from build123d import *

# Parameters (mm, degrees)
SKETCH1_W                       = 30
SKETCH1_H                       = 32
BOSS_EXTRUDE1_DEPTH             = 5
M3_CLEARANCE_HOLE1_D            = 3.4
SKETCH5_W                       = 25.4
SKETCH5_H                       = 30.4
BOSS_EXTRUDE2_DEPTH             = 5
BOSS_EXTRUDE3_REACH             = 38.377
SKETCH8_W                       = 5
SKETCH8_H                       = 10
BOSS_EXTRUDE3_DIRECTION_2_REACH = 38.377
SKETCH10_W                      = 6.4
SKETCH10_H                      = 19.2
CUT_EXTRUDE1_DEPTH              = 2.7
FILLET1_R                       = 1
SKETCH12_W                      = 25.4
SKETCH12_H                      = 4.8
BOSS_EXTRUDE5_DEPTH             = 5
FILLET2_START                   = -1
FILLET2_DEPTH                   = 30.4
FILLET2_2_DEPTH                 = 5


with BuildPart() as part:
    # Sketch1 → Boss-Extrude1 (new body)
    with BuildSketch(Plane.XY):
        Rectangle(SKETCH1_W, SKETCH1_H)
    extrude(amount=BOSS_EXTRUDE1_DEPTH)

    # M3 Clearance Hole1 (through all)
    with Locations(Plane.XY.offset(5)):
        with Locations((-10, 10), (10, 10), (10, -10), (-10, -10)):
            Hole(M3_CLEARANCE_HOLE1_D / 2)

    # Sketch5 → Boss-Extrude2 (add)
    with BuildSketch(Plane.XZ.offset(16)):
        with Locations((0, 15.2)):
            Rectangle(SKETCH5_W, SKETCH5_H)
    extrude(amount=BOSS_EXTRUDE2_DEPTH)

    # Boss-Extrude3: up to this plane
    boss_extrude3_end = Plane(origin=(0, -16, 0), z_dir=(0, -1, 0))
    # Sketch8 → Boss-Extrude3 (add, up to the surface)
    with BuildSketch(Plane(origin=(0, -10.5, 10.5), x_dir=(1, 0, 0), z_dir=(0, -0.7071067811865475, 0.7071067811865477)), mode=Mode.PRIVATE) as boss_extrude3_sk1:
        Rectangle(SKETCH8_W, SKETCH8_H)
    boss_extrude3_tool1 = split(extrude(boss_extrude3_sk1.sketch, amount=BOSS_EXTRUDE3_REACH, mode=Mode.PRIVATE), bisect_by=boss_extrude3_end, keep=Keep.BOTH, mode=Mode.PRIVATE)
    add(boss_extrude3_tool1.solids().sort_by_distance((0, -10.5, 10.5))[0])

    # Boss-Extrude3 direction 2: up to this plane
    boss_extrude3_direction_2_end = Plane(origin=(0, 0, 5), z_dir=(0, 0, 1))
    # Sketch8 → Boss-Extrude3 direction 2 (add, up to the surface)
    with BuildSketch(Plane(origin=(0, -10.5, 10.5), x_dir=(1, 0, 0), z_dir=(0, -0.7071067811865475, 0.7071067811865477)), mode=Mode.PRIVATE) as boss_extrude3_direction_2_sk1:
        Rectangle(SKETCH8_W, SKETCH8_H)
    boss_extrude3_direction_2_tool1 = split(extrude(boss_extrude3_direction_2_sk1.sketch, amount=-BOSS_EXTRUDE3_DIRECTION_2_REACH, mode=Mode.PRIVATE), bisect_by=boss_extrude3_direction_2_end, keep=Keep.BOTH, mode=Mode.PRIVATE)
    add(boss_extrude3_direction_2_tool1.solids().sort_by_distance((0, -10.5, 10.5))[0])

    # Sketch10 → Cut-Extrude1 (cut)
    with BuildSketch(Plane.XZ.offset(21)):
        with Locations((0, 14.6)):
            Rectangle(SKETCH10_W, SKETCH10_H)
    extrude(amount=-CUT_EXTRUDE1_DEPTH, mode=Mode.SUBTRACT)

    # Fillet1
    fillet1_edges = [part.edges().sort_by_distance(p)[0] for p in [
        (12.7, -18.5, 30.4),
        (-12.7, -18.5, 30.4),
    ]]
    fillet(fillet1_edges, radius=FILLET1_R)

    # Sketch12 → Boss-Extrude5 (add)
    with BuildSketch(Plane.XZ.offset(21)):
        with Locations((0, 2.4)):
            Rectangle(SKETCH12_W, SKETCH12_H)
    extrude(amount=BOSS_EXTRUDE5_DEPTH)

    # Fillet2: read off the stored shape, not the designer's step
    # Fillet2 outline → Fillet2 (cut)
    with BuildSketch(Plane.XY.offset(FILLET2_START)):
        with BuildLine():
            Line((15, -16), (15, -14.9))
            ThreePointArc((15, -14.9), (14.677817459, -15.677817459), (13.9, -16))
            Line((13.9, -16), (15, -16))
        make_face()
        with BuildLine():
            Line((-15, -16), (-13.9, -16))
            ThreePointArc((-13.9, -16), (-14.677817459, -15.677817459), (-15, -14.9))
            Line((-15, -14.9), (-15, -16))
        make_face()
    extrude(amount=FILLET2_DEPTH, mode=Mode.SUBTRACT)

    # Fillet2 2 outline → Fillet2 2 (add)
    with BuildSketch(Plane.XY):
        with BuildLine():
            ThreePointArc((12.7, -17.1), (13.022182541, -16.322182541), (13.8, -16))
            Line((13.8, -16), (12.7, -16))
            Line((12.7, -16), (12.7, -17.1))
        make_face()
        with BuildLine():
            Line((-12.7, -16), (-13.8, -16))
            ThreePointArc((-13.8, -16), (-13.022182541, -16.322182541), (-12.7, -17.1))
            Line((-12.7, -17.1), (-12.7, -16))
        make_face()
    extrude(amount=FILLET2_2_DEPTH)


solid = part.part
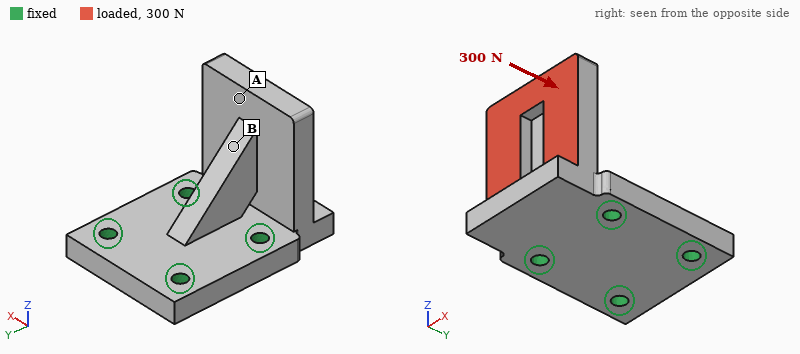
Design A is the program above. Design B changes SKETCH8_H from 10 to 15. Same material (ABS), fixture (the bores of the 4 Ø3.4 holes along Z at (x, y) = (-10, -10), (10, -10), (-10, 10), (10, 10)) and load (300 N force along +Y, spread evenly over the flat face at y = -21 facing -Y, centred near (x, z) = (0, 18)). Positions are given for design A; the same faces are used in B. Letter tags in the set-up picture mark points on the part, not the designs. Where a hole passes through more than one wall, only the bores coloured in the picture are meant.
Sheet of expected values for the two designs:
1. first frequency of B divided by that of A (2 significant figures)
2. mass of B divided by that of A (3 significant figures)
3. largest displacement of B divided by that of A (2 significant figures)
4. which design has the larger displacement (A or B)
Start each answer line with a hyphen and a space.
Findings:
- 1.1
- 1.04
- 0.70
- A
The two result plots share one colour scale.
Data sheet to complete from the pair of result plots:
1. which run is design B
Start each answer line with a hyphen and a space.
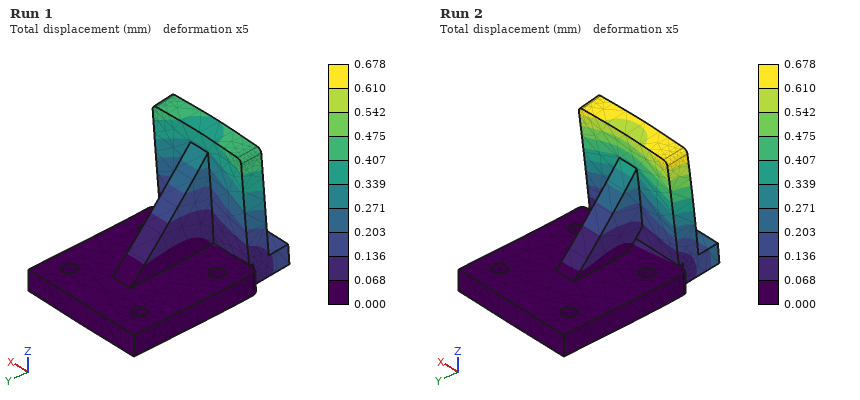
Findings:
- Run 1
